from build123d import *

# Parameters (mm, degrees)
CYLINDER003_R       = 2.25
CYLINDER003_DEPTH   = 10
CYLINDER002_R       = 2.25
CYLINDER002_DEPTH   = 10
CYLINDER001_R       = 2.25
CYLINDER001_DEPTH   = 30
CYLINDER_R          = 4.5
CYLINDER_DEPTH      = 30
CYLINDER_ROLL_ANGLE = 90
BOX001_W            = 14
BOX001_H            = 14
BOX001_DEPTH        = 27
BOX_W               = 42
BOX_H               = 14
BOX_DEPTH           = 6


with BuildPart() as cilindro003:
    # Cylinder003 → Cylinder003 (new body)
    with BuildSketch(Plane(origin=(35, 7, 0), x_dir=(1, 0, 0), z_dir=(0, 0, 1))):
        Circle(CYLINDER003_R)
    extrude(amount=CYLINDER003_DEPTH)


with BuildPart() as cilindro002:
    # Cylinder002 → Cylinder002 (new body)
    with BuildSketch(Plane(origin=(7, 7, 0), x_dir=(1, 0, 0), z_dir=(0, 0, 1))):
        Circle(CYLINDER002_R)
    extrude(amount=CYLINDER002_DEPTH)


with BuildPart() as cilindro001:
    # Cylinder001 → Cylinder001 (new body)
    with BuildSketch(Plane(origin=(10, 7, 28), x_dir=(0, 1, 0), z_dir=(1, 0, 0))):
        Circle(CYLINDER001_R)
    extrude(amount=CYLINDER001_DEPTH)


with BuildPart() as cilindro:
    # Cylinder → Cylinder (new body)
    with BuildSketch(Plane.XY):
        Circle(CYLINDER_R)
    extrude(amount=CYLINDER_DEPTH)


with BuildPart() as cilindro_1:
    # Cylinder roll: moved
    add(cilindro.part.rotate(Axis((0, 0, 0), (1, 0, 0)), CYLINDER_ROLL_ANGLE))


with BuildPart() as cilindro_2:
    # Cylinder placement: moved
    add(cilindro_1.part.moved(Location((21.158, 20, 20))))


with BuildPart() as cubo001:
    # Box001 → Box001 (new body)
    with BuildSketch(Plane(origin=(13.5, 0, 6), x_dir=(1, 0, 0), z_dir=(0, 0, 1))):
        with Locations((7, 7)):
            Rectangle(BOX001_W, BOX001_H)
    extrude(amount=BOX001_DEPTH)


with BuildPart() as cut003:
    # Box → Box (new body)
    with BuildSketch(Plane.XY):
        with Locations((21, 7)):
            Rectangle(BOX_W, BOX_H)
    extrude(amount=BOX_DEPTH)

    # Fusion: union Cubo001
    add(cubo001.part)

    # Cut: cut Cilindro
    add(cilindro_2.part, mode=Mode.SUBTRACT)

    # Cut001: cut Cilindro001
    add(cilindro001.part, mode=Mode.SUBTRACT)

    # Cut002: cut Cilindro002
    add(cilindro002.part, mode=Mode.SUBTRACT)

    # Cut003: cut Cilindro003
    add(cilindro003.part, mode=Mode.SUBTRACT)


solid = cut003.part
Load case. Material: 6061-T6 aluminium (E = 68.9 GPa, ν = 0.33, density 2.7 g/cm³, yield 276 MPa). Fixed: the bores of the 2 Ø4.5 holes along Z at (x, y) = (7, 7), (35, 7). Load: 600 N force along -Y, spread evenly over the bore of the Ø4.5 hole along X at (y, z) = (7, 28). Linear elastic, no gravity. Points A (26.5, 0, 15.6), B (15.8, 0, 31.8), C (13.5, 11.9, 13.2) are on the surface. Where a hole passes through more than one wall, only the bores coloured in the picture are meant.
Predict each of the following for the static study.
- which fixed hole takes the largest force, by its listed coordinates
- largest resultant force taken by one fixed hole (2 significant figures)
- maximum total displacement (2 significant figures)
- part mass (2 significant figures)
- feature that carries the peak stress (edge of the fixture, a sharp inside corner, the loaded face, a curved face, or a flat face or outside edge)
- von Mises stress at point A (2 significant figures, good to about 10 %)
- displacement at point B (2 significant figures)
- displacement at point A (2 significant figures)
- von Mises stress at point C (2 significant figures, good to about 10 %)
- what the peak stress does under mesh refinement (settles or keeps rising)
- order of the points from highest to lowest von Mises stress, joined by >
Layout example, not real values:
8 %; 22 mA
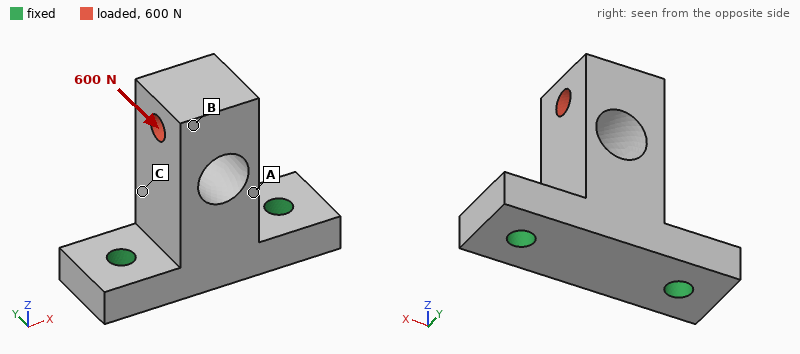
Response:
(7, 7); 320 N; 0.11 mm; 20 g; edge of the fixture; 36 MPa; 0.10 mm; 0.045 mm; 24 MPa; keeps rising; A > C > B
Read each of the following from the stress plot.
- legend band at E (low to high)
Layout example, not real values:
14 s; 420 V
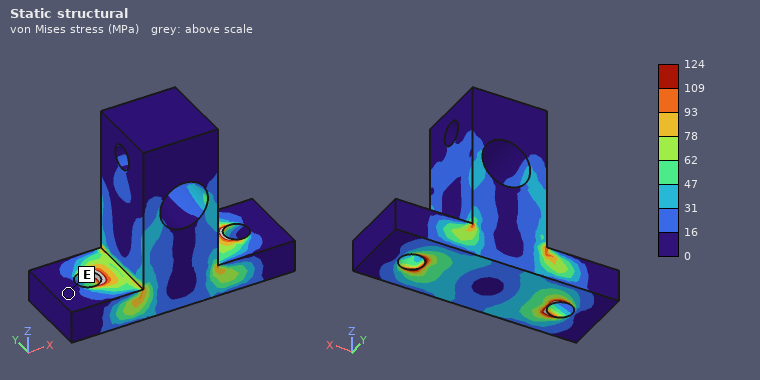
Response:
0 to 16 MPa
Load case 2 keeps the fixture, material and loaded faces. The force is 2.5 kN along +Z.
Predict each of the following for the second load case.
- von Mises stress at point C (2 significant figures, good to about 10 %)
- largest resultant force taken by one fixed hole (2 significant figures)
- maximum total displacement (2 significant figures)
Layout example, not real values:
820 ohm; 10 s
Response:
26 MPa; 1.3 kN; 23 µm
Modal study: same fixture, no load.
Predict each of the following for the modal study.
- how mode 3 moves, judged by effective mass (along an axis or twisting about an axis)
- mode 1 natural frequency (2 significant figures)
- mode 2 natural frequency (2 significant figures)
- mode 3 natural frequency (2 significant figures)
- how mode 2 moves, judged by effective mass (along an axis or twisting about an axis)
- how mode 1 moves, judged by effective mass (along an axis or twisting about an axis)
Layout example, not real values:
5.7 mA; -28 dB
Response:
along Z; 5400 Hz; 8700 Hz; 19 kHz; along X; along Y
